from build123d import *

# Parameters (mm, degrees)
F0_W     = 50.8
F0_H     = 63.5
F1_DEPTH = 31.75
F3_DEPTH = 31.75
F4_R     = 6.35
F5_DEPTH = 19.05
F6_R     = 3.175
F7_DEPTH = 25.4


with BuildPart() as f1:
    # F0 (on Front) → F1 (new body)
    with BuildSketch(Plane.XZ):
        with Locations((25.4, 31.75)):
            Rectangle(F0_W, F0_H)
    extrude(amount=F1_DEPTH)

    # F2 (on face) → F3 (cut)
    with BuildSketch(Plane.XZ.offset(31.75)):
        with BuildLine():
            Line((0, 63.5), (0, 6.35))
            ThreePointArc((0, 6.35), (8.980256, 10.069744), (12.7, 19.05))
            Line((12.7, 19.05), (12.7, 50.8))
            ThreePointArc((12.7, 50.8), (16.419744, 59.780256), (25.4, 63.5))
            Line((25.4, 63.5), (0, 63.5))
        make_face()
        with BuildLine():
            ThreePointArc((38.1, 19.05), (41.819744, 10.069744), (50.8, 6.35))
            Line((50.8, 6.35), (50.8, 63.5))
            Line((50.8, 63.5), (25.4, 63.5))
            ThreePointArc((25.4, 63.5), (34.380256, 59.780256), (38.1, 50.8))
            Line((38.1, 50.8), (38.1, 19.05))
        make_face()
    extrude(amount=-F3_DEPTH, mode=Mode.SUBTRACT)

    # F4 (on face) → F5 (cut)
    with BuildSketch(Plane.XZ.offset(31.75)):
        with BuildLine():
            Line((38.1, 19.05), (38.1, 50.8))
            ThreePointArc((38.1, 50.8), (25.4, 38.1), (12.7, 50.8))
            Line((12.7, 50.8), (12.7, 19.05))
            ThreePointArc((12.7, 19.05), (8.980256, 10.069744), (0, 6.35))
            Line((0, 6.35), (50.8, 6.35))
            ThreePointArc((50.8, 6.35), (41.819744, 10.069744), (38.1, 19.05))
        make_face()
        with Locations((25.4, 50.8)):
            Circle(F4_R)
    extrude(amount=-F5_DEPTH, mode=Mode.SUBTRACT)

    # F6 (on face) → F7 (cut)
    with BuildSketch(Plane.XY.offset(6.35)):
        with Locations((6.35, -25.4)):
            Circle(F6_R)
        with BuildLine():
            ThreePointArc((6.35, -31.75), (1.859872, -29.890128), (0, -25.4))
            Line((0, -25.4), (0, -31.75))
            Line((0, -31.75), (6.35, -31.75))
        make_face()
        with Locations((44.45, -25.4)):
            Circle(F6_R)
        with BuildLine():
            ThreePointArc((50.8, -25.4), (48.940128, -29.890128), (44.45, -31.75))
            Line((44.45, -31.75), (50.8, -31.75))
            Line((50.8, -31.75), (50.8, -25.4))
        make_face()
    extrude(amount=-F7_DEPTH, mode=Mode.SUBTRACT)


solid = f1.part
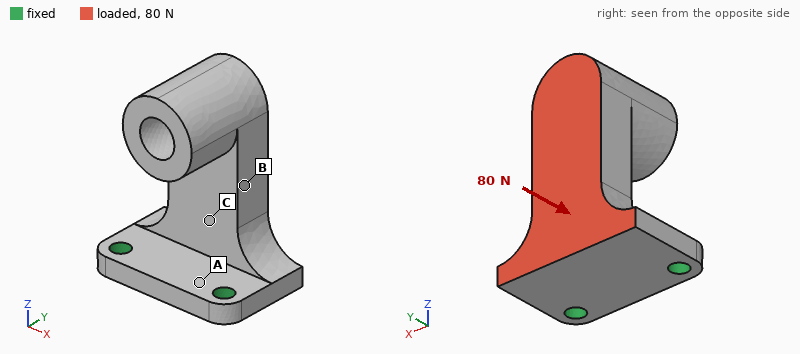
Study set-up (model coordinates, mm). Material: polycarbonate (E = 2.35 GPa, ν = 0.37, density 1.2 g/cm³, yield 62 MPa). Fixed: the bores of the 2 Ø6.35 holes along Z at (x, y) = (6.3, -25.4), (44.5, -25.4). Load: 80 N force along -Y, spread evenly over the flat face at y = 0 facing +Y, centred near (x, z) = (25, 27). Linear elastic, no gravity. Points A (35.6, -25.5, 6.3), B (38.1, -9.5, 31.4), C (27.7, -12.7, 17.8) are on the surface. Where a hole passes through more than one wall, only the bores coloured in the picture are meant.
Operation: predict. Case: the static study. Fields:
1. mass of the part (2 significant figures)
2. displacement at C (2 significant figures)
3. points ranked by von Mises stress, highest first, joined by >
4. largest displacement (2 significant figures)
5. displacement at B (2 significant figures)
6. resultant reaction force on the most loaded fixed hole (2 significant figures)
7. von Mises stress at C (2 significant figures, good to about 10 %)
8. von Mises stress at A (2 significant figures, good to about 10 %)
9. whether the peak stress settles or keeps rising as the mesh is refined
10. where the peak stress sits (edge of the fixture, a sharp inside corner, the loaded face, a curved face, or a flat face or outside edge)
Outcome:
42 g
0.20 mm
A > C > B
0.89 mm
0.39 mm
45 N
1.6 MPa
2.8 MPa
keeps rising
edge of the fixture
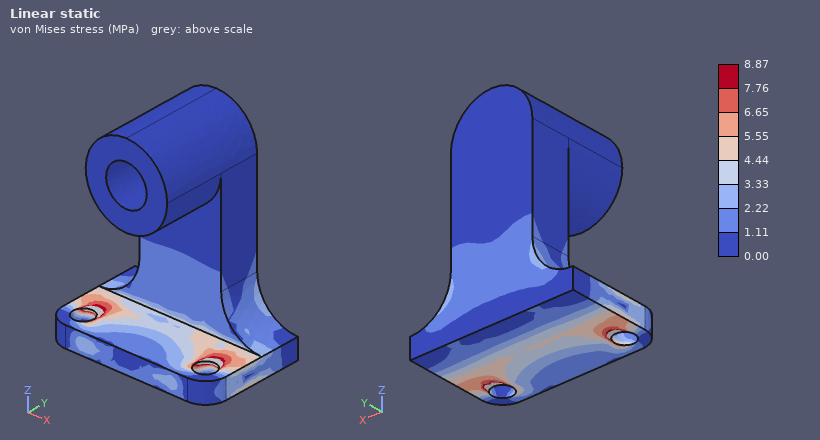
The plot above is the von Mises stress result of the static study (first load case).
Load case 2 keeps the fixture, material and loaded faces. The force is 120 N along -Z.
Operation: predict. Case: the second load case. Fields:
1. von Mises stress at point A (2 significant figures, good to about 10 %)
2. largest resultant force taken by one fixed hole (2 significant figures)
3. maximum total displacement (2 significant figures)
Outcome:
3.7 MPa
60 N
0.90 mm
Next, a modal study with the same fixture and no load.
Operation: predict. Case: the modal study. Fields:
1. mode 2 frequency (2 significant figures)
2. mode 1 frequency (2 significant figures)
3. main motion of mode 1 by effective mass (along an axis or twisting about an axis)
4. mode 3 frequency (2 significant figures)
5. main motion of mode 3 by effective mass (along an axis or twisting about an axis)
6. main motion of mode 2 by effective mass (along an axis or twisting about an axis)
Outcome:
610 Hz
260 Hz
along Y
1200 Hz
along Z
along X
